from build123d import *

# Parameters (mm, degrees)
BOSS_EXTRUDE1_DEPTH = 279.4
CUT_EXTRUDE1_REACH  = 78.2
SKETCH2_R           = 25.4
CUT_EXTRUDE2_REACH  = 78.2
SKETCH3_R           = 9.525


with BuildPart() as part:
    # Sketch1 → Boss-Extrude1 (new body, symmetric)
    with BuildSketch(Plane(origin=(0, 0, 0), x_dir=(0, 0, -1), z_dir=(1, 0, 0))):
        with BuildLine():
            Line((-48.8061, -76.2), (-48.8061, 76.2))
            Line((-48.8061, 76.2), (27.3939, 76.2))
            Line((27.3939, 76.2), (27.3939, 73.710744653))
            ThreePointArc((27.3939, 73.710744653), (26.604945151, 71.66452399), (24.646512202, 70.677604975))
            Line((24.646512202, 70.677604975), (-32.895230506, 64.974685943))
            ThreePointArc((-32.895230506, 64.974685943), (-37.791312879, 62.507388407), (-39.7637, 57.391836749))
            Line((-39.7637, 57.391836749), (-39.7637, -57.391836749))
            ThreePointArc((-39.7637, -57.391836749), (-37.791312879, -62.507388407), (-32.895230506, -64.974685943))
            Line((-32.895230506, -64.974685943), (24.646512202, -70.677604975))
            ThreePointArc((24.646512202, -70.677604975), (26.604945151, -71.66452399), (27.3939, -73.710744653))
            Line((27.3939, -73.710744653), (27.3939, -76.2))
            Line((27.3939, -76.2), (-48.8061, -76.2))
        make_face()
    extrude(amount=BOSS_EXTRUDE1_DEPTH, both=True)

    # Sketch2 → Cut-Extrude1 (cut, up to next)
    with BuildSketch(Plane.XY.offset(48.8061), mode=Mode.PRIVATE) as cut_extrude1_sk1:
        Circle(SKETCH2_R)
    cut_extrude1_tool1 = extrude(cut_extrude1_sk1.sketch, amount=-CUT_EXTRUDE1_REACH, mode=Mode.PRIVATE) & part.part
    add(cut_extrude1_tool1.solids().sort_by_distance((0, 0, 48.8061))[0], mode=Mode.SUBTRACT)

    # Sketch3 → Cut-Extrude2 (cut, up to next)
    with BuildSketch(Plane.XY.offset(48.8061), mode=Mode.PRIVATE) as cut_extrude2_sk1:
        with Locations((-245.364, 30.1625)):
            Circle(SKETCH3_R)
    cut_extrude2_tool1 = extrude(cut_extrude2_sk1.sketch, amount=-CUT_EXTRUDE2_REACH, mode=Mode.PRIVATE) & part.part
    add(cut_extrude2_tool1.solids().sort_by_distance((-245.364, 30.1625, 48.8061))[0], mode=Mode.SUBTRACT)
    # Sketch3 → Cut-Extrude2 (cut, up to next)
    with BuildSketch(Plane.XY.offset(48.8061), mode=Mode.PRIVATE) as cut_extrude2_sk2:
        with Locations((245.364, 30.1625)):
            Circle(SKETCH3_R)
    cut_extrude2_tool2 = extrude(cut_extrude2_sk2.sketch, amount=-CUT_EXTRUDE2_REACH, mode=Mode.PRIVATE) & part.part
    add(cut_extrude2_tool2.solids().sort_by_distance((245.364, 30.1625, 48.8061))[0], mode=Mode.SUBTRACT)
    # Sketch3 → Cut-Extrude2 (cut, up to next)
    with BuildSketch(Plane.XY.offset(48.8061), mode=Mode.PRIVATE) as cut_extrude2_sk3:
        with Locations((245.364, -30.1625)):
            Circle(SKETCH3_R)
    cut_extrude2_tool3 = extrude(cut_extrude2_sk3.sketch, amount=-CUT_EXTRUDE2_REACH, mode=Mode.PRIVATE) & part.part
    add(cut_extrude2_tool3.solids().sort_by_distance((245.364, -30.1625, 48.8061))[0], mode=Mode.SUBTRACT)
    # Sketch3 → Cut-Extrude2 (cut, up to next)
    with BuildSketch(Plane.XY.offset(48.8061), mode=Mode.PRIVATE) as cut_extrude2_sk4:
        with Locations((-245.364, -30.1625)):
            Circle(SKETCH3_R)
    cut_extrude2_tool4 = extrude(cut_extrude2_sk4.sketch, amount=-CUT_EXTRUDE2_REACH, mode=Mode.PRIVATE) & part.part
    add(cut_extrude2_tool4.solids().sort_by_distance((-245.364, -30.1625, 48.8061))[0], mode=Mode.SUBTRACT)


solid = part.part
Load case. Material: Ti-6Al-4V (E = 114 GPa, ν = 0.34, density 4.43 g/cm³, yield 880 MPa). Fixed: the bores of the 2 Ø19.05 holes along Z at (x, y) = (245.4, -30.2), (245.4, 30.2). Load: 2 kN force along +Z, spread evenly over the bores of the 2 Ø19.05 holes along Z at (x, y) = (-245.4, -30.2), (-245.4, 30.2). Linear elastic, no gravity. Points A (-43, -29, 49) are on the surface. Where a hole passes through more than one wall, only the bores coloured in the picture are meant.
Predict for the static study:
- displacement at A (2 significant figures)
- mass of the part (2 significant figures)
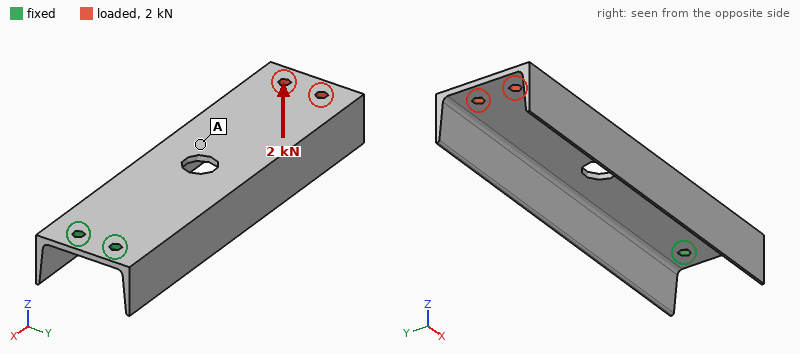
3.2 mm
6.2 kg
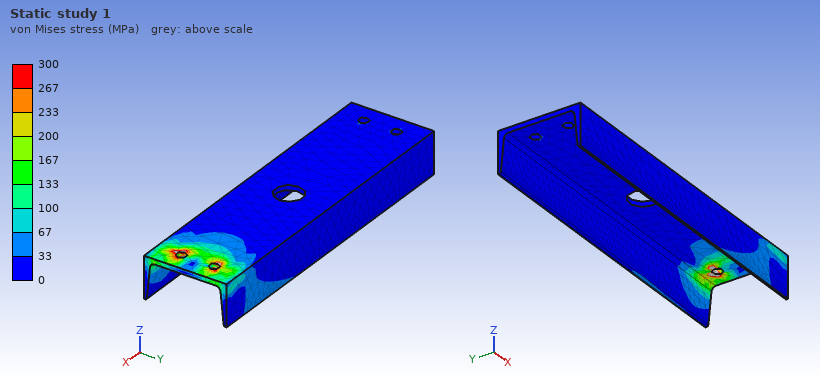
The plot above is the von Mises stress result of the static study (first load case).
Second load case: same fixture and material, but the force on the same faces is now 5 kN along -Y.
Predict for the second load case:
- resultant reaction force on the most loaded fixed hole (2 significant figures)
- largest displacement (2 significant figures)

32 kN
0.79 mm
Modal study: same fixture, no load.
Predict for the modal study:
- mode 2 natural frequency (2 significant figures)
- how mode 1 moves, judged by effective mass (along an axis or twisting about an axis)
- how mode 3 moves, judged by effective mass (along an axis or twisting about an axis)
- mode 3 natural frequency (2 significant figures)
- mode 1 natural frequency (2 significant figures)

140 Hz
along Z
along Y
310 Hz
65 Hz
